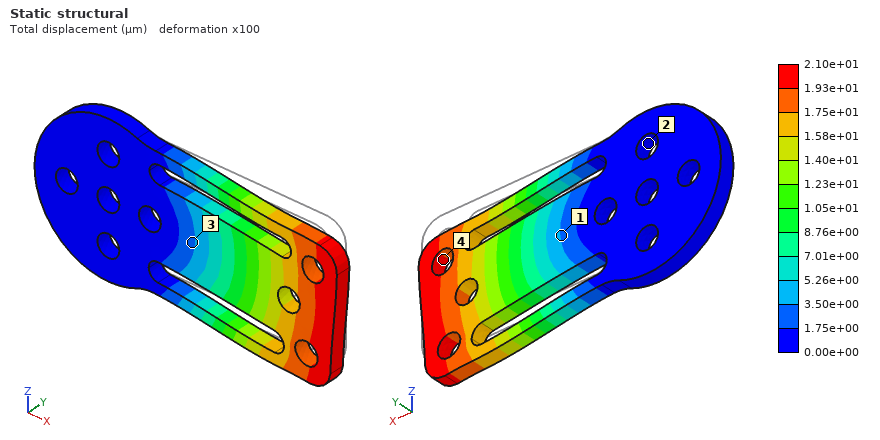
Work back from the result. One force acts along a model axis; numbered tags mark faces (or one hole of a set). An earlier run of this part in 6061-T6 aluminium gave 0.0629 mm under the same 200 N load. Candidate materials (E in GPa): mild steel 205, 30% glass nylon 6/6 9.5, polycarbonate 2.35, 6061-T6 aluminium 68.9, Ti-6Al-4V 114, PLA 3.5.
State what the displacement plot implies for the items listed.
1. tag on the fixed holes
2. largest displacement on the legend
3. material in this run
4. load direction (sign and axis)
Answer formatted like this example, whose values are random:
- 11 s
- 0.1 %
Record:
- 2
- 2.10e+01 µm
- mild steel
- -Z
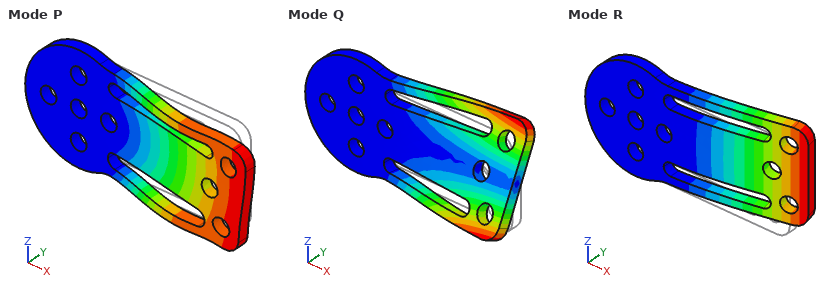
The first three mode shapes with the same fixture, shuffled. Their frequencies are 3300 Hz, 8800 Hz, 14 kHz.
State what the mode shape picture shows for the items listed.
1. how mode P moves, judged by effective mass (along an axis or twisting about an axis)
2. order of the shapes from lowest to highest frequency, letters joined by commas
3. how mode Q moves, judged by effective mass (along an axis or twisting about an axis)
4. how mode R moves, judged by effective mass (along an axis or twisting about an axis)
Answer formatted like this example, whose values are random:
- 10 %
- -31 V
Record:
- along Z
- R, Q, P
- twisting about X
- along Y
